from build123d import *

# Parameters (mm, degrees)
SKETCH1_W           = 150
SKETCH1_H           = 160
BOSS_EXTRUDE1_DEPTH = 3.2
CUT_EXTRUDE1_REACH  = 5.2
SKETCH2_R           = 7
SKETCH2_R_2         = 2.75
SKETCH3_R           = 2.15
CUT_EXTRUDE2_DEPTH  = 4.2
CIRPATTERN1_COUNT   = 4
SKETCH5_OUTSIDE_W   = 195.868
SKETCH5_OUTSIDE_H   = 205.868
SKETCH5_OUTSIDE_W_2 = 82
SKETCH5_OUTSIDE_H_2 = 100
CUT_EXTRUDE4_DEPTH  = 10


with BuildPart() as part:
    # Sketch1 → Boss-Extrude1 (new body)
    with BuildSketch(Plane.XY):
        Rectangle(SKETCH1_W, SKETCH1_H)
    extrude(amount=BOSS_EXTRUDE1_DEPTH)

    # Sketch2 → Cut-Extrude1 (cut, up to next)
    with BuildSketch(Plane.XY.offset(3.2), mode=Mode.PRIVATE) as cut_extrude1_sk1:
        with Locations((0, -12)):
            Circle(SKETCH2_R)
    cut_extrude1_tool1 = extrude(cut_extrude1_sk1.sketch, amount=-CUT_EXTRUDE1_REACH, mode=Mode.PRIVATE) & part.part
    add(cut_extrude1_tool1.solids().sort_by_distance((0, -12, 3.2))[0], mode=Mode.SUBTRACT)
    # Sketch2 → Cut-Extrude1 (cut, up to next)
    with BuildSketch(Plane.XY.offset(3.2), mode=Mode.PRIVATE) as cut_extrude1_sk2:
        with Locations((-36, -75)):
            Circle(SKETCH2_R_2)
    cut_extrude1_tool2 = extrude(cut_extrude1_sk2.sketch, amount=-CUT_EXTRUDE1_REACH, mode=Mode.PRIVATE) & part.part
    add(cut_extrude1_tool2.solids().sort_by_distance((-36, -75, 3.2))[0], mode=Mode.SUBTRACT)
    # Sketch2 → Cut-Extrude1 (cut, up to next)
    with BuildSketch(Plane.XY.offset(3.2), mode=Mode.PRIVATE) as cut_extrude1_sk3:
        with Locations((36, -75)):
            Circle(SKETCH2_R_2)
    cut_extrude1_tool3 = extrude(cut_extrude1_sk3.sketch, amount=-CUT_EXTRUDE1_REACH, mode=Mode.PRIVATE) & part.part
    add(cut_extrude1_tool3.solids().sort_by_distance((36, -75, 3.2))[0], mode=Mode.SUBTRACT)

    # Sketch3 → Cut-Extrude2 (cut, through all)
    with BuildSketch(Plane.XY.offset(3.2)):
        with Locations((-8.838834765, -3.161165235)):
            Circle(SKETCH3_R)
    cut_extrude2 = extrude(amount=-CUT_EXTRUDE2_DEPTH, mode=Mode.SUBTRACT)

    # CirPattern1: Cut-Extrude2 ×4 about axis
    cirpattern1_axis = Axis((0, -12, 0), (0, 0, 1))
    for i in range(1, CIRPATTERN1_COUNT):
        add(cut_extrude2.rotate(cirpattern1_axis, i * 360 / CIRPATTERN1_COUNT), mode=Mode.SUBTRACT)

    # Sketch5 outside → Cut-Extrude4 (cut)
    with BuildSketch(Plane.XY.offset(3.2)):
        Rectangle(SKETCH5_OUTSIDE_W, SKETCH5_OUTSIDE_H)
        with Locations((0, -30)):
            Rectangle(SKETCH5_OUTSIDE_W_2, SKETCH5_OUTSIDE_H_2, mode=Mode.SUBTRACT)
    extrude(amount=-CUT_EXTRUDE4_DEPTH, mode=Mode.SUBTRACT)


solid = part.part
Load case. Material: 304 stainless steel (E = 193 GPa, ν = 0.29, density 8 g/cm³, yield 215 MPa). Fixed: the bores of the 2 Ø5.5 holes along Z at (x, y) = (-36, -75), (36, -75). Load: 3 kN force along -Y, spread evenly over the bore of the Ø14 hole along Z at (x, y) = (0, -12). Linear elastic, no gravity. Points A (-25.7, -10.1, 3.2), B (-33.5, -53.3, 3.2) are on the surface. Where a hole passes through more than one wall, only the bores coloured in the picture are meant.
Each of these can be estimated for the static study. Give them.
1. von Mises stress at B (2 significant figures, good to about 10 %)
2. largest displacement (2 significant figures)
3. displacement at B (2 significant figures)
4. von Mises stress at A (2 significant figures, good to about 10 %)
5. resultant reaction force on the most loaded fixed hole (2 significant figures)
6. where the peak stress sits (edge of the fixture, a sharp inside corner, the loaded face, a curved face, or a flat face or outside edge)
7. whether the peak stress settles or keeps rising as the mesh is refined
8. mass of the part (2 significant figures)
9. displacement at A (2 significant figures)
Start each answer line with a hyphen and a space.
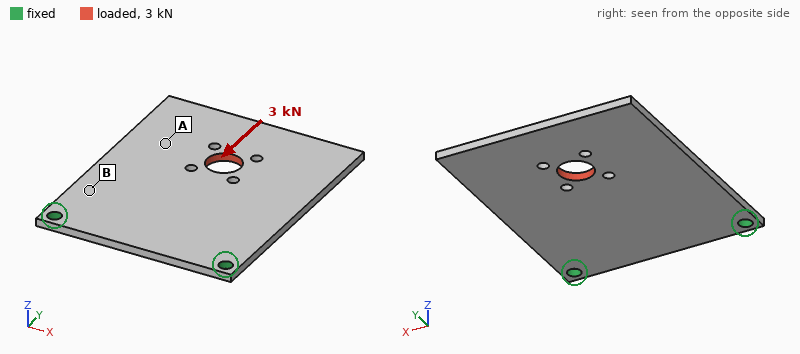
- 19 MPa
- 8.8 µm
- 2.9 µm
- 7.0 MPa
- 1.6 kN
- edge of the fixture
- keeps rising
- 200 g
- 5.6 µm
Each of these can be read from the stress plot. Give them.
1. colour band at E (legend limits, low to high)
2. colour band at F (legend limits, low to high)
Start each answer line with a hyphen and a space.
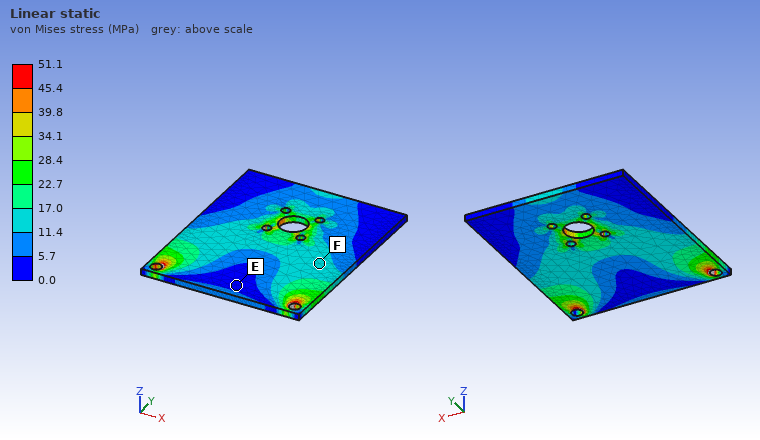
- 0.0 to 5.7 MPa
- 11.4 to 17.0 MPa
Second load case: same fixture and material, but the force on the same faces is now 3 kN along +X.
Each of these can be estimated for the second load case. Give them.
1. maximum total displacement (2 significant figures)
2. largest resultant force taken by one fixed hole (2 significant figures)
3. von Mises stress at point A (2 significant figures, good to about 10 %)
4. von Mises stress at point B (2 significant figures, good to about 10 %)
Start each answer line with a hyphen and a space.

- 32 µm
- 3.0 kN
- 11 MPa
- 34 MPa
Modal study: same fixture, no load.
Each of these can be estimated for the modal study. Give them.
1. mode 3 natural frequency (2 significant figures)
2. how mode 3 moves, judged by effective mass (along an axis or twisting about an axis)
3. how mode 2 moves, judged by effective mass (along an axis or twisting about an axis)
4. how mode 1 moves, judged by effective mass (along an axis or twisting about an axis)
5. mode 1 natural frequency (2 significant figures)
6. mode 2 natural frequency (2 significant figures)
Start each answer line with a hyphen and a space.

- 1500 Hz
- along Z
- twisting about Y
- along Z
- 240 Hz
- 780 Hz
